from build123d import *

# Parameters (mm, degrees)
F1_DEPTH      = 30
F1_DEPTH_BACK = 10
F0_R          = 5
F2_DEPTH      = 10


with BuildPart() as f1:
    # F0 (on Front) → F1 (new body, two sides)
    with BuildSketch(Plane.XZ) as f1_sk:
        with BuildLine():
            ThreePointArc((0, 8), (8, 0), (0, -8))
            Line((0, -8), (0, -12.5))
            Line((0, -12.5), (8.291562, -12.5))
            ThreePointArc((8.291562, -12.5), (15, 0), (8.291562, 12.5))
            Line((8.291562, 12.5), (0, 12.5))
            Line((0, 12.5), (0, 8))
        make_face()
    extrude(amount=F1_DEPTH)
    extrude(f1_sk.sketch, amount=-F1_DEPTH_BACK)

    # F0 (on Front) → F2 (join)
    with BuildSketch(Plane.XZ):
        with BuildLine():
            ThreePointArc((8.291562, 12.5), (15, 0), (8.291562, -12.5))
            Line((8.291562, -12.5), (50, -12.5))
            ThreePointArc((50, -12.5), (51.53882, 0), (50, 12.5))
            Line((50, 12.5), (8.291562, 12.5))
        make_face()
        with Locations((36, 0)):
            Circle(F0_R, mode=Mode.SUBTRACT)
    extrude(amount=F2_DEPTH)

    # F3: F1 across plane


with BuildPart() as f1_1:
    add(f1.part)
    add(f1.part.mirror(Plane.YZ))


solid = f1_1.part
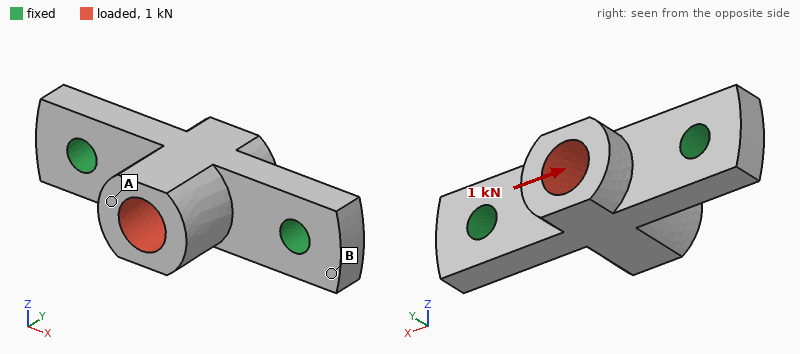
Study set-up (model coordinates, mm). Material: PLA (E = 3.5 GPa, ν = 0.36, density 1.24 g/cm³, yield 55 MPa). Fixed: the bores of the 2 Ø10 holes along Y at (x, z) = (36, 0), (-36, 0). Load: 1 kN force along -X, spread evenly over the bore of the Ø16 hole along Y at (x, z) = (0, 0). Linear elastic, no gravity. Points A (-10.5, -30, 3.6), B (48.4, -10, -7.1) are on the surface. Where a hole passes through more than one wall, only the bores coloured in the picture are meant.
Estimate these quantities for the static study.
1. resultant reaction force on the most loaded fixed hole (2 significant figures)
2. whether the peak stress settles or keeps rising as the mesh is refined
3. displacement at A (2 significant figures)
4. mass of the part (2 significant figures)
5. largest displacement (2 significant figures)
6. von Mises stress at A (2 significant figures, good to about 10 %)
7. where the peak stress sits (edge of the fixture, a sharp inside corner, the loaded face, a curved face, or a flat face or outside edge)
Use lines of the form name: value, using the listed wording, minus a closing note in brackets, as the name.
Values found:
resultant reaction force on the most loaded fixed hole: 510 N
whether the peak stress settles or keeps rising as the mesh is refined: keeps rising
displacement at A: 58 µm
mass of the part: 44 g
largest displacement: 60 µm
von Mises stress at A: 1.0 MPa
where the peak stress sits: edge of the fixture
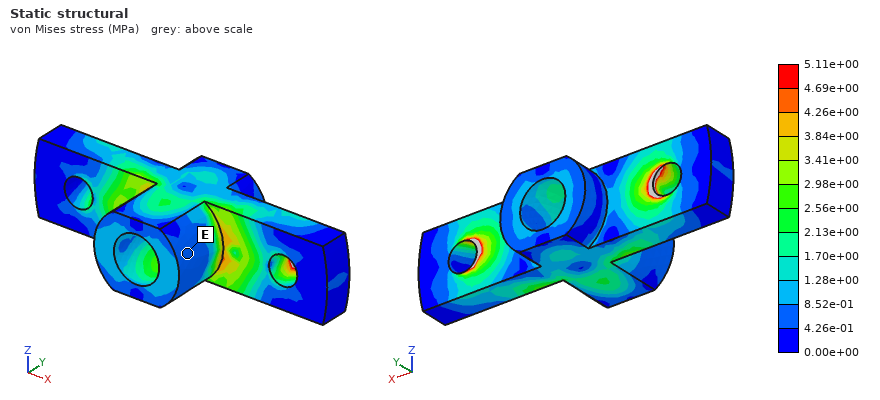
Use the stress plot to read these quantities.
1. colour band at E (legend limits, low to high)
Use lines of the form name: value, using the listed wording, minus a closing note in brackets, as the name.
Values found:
colour band at E: 4.26e-01 to 8.52e-01 MPa
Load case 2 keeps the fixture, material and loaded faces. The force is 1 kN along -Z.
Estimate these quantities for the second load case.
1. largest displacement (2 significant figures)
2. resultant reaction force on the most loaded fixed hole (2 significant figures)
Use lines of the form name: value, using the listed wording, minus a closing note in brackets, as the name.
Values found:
largest displacement: 0.26 mm
resultant reaction force on the most loaded fixed hole: 500 N
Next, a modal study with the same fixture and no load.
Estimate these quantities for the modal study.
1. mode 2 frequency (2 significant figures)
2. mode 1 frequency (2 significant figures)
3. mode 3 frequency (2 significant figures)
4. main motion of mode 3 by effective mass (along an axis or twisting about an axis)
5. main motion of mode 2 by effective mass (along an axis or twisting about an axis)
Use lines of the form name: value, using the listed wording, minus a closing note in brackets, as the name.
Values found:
mode 2 frequency: 2900 Hz
mode 1 frequency: 2000 Hz
mode 3 frequency: 3700 Hz
main motion of mode 3 by effective mass: along Z
main motion of mode 2 by effective mass: along Y
